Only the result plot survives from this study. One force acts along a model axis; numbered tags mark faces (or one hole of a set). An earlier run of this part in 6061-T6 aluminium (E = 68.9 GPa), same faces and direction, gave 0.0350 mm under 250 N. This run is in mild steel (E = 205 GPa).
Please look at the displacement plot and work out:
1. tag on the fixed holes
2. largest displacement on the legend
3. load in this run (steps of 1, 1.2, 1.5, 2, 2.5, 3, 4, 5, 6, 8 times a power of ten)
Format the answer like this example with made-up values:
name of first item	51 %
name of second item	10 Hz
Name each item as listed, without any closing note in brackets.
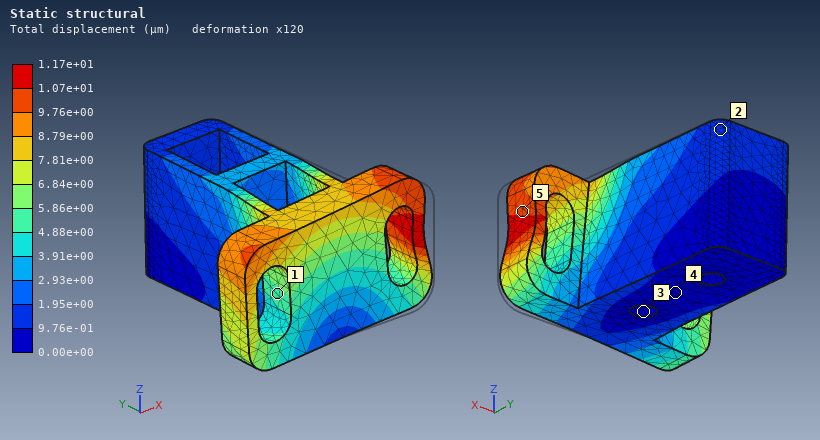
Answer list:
tag on the fixed holes	3
largest displacement on the legend	1.17e+01 µm
load in this run	250 N
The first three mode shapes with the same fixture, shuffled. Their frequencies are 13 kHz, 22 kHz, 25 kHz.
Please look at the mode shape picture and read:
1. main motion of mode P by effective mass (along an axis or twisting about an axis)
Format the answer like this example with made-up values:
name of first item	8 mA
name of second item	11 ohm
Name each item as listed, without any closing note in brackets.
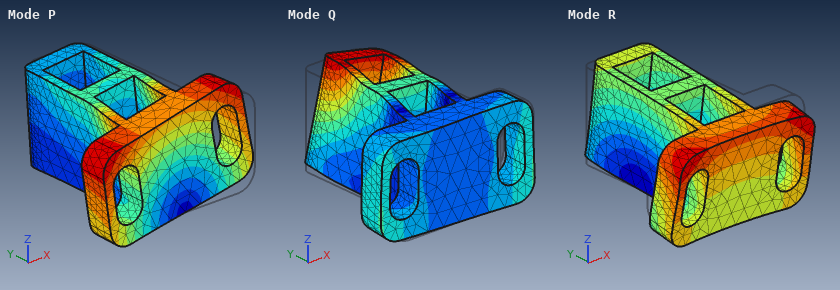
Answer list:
main motion of mode P by effective mass	along X
